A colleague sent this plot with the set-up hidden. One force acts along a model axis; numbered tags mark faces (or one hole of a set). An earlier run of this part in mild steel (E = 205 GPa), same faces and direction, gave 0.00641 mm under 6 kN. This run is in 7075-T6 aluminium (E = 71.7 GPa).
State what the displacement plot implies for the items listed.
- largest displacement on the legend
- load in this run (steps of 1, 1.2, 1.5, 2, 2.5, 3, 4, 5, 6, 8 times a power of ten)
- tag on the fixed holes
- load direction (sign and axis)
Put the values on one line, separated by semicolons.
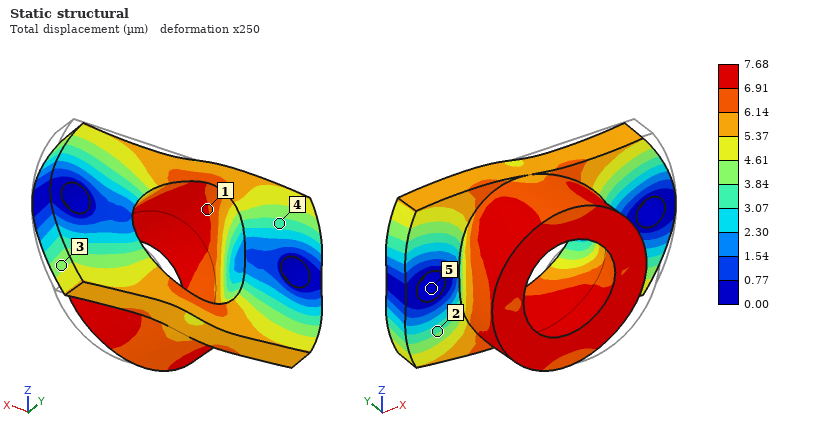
7.68 µm; 2.5 kN; 5; -X
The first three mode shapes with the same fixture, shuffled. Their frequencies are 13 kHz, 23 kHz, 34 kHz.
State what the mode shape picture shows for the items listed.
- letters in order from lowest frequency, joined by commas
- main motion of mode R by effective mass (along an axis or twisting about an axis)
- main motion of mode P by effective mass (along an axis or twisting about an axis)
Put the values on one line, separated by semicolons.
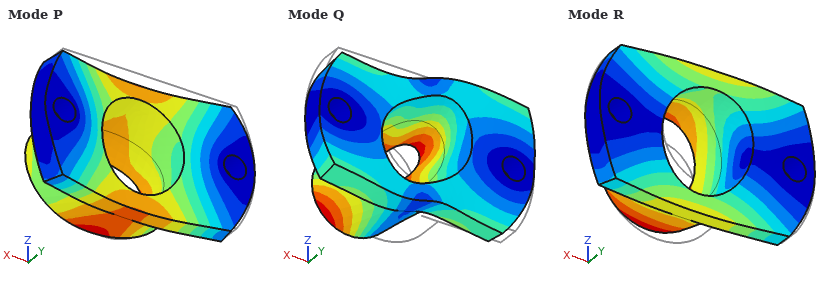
R, P, Q; along Z; along Y
